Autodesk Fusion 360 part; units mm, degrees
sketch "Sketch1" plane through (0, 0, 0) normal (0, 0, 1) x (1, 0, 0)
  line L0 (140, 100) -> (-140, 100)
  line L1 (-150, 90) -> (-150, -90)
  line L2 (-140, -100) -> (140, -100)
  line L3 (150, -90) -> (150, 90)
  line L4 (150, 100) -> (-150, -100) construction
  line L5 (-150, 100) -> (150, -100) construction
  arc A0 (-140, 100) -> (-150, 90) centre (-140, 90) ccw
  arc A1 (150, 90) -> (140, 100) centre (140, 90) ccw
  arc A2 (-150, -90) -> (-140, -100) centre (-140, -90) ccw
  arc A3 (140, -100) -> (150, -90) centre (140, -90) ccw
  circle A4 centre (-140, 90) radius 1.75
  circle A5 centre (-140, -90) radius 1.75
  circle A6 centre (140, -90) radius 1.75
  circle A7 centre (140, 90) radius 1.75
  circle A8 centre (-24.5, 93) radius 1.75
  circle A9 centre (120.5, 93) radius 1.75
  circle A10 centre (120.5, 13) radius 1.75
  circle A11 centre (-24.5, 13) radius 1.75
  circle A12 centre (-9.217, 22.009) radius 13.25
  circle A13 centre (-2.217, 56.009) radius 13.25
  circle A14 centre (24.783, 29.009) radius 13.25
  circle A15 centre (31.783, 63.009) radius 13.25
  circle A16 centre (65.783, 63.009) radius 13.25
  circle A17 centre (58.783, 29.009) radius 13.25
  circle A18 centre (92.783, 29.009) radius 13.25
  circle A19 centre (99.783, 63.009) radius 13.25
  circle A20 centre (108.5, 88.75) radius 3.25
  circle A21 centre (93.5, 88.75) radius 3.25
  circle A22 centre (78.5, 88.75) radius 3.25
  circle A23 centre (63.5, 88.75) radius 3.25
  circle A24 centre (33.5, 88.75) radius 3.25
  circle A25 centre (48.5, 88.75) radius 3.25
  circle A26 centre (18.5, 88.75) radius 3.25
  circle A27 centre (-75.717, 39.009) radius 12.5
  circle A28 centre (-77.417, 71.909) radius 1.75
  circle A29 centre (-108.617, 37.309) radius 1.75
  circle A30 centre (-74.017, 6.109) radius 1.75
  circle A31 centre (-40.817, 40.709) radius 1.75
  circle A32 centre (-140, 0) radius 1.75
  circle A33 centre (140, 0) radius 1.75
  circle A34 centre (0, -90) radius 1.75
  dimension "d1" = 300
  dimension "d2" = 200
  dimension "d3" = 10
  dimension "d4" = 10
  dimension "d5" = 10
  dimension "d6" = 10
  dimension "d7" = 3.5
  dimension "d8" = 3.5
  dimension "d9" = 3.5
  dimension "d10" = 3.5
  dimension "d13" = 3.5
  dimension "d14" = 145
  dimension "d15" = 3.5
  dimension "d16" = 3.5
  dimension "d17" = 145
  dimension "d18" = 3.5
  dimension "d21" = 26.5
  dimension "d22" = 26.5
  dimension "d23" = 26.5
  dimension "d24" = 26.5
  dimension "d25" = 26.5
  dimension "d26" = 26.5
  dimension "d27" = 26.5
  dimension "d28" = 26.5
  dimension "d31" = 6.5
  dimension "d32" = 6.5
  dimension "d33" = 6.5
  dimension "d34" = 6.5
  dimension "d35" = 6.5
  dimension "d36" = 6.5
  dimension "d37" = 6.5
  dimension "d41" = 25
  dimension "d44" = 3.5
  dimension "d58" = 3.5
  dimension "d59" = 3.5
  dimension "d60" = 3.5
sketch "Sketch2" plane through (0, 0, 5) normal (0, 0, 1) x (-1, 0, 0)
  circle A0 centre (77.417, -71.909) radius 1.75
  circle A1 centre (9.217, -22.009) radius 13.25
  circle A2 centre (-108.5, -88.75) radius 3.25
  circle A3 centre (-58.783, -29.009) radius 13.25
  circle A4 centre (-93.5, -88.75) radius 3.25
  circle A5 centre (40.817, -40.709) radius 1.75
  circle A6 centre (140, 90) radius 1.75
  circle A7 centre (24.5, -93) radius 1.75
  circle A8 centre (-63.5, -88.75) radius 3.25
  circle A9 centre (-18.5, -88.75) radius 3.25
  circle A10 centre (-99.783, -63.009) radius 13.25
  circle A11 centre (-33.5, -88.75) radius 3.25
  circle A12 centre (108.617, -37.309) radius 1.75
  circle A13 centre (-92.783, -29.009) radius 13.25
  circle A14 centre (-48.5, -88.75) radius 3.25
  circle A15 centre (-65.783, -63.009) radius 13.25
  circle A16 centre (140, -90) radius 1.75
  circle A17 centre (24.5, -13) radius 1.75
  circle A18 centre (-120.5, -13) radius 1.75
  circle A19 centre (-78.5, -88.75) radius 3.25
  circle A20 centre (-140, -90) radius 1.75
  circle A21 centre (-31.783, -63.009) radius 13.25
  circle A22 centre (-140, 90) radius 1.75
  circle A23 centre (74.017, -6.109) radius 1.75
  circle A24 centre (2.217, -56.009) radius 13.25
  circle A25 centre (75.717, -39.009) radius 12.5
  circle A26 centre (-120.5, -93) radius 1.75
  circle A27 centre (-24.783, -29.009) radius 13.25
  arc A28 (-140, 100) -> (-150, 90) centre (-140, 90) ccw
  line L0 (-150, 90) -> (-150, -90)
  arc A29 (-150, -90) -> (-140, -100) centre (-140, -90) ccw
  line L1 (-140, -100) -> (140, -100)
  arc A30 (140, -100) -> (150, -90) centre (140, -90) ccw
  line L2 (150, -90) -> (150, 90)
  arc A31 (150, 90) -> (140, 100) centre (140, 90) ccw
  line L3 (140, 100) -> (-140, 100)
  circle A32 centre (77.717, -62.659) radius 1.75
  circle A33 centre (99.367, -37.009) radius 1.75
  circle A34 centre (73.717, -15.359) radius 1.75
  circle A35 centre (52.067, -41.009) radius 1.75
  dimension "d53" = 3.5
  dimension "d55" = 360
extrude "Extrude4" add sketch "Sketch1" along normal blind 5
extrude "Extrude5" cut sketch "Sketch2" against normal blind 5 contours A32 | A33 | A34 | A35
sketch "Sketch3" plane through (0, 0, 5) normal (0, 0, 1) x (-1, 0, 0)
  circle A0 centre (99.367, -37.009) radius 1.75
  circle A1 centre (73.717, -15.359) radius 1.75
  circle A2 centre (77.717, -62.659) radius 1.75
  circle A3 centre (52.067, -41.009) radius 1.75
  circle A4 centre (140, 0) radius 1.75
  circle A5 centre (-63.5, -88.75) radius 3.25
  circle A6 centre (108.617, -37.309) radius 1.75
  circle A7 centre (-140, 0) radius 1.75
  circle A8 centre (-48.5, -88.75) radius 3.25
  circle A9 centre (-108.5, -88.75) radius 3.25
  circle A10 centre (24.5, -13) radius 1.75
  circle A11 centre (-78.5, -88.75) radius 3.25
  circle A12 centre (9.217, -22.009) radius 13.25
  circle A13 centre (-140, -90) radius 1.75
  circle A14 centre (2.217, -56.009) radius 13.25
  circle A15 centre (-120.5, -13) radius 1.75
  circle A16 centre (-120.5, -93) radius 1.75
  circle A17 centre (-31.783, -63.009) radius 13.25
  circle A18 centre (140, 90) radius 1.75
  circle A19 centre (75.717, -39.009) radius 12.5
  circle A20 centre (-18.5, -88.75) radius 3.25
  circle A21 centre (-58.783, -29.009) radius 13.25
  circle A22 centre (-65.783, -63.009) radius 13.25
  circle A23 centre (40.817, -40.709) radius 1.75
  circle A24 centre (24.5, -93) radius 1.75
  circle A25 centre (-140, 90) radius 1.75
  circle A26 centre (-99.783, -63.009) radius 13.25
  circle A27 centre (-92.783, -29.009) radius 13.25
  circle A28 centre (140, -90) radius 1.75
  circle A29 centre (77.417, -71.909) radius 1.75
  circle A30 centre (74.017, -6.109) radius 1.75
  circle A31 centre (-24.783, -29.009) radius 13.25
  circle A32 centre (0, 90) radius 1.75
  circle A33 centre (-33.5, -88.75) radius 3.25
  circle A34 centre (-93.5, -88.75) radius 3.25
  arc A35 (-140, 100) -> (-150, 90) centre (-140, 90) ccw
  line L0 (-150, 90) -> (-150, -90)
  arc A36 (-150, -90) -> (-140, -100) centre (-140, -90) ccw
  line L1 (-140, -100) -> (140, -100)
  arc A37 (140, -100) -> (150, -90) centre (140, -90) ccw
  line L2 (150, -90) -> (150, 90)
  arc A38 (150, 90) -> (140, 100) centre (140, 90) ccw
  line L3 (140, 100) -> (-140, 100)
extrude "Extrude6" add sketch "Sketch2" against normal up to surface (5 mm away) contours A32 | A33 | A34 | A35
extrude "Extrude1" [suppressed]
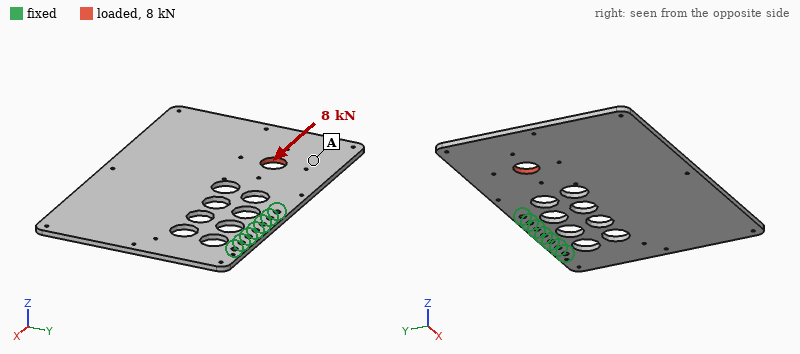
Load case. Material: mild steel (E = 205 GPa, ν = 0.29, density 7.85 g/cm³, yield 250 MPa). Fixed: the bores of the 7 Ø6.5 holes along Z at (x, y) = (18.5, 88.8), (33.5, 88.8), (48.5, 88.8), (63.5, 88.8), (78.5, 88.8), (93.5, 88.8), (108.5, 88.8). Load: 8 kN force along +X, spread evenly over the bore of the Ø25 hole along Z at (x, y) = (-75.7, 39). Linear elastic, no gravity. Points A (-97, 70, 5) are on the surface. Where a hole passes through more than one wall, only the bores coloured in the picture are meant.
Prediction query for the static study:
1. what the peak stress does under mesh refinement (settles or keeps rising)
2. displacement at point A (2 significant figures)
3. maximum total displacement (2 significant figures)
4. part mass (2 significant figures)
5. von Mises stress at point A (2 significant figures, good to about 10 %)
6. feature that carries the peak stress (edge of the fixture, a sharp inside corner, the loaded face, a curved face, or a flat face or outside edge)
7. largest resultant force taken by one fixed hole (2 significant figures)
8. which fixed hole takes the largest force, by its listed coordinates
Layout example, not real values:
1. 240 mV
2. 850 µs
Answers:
1. keeps rising
2. 0.064 mm
3. 0.11 mm
4. 2.1 kg
5. 12 MPa
6. edge of the fixture
7. 5.6 kN
8. (18.5, 88.8)
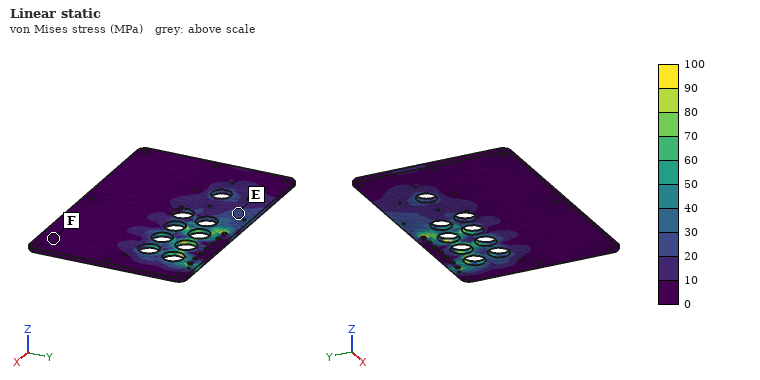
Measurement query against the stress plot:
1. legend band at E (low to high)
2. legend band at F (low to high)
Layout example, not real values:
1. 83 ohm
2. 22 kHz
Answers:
1. 20 to 30 MPa
2. 0 to 10 MPa
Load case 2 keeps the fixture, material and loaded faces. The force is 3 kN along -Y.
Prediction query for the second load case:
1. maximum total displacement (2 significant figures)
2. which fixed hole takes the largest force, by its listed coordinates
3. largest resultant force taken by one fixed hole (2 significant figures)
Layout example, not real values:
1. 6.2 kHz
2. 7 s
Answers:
1. 0.10 mm
2. (18.5, 88.8)
3. 5.7 kN
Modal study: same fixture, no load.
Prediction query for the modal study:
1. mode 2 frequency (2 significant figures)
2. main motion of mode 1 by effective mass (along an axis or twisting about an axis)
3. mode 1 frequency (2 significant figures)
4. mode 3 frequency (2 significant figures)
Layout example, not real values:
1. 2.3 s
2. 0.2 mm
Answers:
1. 110 Hz
2. along Z
3. 62 Hz
4. 250 Hz
